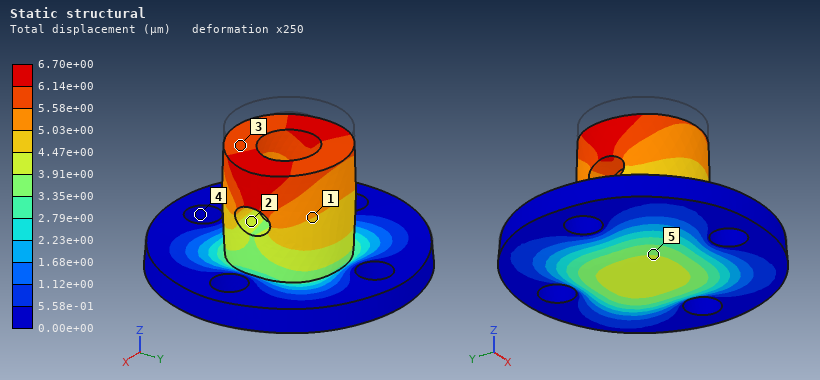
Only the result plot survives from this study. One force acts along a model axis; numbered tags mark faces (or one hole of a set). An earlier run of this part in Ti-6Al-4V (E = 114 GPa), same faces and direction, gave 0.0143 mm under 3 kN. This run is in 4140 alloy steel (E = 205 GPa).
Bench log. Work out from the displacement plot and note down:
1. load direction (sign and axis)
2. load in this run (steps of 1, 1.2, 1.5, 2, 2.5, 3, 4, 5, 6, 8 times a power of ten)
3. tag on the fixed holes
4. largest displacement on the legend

-Z
2.5 kN
4
6.70e+00 µm
